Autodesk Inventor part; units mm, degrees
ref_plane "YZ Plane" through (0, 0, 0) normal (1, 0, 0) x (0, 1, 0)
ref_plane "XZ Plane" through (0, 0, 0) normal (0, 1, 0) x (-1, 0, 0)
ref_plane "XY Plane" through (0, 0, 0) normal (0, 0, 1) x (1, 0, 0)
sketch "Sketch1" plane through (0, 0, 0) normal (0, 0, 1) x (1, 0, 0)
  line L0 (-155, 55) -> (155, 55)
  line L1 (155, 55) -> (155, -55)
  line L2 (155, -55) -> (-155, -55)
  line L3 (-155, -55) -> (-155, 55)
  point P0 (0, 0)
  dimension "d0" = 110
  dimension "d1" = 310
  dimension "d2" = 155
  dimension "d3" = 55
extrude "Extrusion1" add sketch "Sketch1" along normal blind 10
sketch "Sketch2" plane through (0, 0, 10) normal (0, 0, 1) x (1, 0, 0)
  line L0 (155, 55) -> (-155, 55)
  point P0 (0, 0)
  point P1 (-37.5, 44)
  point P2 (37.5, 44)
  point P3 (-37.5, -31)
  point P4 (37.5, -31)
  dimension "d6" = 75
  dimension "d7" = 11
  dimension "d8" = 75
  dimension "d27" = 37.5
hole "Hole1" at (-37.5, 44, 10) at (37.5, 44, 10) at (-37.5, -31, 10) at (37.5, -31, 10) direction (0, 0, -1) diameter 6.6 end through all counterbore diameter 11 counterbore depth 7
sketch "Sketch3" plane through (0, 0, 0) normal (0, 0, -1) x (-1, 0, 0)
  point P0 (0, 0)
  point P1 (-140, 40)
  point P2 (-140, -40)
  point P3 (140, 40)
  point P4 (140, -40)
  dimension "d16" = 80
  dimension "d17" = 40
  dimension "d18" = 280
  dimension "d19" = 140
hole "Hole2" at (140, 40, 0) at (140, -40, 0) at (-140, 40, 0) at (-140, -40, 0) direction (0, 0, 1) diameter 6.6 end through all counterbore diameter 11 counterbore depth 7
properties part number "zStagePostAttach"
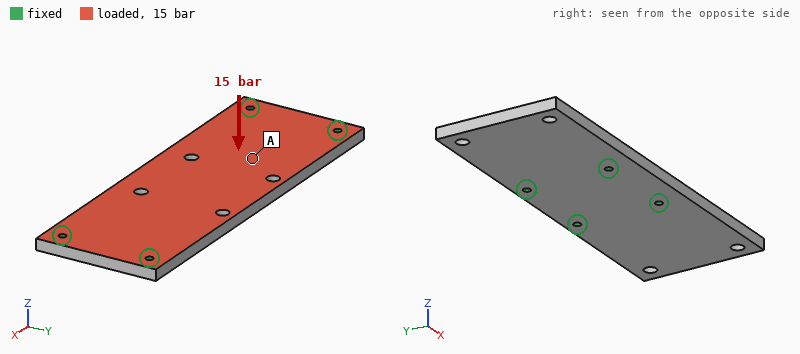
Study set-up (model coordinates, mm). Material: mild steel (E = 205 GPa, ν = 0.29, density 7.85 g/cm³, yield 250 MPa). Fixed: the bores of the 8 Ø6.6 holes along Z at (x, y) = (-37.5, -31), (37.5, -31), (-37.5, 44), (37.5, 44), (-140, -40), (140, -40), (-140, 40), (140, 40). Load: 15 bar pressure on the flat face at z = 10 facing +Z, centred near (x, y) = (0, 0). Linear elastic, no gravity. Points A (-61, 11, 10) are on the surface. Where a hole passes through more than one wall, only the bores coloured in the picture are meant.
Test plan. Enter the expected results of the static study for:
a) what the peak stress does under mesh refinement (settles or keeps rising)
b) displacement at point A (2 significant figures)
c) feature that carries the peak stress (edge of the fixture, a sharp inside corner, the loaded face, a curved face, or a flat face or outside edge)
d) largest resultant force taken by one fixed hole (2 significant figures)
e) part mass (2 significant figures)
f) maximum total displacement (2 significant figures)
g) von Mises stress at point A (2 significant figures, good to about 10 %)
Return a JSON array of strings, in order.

["keeps rising", "52 µm", "edge of the fixture", "9.2 kN", "2.6 kg", "69 µm", "34 MPa"]
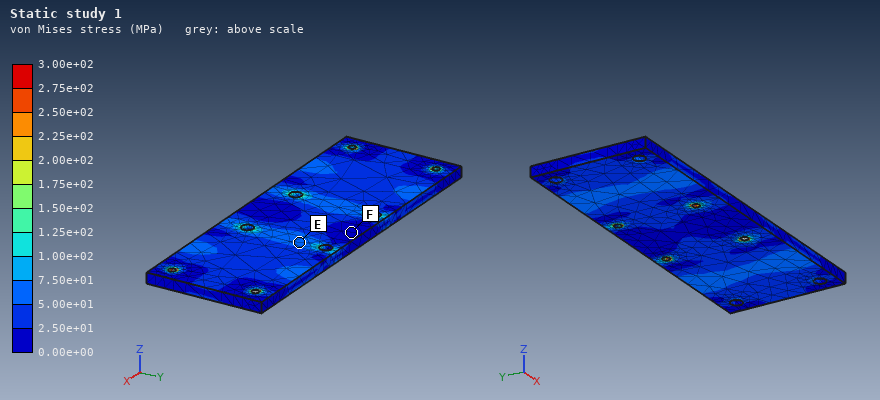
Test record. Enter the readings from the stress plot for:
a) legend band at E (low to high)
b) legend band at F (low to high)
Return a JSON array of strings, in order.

["5.00e+01 to 7.50e+01 MPa", "0.00e+00 to 2.50e+01 MPa"]
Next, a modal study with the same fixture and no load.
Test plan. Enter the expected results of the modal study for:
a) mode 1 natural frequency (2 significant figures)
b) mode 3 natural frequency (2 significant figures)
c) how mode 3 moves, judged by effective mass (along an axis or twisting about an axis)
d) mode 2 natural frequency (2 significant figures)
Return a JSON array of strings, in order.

["2900 Hz", "4100 Hz", "twisting about X", "2900 Hz"]
